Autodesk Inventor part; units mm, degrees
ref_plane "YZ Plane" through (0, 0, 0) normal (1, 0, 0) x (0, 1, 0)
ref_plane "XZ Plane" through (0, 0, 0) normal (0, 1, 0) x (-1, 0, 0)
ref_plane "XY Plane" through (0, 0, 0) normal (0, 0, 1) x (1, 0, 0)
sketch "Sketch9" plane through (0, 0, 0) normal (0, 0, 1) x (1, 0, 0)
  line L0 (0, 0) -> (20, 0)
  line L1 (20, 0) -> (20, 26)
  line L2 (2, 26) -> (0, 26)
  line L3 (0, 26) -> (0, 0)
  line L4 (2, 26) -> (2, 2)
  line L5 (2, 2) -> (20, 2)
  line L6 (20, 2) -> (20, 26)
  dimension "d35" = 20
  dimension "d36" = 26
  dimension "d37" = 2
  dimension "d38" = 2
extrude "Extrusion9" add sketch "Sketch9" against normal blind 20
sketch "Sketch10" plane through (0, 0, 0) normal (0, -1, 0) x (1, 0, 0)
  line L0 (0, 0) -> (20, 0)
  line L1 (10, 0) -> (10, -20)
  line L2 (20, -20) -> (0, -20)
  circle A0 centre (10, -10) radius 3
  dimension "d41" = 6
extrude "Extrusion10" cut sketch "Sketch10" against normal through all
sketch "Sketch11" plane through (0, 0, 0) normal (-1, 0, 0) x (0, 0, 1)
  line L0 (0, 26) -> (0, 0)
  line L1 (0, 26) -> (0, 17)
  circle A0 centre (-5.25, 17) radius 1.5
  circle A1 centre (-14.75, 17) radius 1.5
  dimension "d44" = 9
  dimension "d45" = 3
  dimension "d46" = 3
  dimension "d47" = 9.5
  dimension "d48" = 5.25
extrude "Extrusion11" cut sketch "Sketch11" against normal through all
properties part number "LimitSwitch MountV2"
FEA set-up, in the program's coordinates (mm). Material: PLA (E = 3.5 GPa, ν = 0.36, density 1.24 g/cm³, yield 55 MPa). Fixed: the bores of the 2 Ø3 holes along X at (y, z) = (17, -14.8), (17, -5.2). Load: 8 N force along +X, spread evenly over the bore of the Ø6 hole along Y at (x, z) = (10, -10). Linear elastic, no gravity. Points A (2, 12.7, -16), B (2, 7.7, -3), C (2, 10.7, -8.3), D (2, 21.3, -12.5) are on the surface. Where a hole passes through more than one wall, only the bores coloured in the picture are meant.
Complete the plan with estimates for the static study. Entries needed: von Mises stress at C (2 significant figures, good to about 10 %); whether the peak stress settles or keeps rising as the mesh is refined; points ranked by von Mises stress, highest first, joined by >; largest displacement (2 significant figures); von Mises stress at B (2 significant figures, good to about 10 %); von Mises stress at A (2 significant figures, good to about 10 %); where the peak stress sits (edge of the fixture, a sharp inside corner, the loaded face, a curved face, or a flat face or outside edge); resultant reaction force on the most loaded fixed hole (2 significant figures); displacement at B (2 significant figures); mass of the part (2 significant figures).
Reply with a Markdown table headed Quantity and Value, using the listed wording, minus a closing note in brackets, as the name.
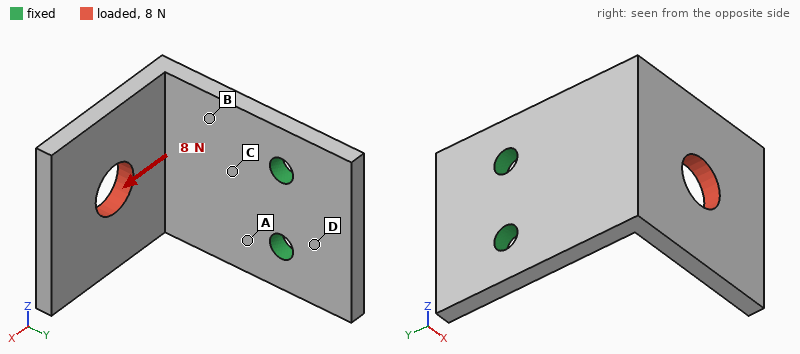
| Quantity | Value |
|---|---|
| von Mises stress at C | 5.2 MPa |
| whether the peak stress settles or keeps rising as the mesh is refined | keeps rising |
| points ranked by von Mises stress, highest first, joined by > | A > C > B > D |
| largest displacement | 0.42 mm |
| von Mises stress at B | 3.8 MPa |
| von Mises stress at A | 6.5 MPa |
| where the peak stress sits | edge of the fixture |
| resultant reaction force on the most loaded fixed hole | 4.0 N |
| displacement at B | 0.076 mm |
| mass of the part | 2.1 g |
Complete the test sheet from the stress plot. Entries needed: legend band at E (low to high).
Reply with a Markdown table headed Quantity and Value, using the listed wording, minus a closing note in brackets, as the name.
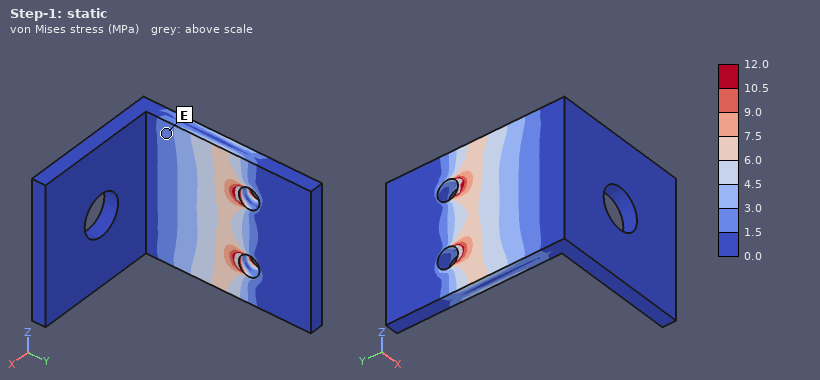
| Quantity | Value |
|---|---|
| legend band at E | 1.5 to 3.0 MPa |
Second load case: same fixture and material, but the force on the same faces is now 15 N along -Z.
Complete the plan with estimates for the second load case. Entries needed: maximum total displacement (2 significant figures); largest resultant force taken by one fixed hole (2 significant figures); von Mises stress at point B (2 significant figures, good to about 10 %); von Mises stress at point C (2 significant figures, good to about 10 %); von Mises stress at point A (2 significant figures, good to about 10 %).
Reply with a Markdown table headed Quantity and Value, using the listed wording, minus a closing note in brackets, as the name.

| Quantity | Value |
|---|---|
| maximum total displacement | 0.41 mm |
| largest resultant force taken by one fixed hole | 24 N |
| von Mises stress at point B | 6.6 MPa |
| von Mises stress at point C | 7.2 MPa |
| von Mises stress at point A | 5.8 MPa |
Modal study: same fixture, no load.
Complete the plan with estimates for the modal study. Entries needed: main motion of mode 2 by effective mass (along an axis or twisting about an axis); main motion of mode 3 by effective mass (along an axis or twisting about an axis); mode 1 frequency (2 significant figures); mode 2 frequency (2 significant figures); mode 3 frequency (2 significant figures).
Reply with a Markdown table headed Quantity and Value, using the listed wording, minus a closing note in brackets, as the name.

| Quantity | Value |
|---|---|
| main motion of mode 2 by effective mass | along Z |
| main motion of mode 3 by effective mass | along X |
| mode 1 frequency | 650 Hz |
| mode 2 frequency | 1100 Hz |
| mode 3 frequency | 1800 Hz |
